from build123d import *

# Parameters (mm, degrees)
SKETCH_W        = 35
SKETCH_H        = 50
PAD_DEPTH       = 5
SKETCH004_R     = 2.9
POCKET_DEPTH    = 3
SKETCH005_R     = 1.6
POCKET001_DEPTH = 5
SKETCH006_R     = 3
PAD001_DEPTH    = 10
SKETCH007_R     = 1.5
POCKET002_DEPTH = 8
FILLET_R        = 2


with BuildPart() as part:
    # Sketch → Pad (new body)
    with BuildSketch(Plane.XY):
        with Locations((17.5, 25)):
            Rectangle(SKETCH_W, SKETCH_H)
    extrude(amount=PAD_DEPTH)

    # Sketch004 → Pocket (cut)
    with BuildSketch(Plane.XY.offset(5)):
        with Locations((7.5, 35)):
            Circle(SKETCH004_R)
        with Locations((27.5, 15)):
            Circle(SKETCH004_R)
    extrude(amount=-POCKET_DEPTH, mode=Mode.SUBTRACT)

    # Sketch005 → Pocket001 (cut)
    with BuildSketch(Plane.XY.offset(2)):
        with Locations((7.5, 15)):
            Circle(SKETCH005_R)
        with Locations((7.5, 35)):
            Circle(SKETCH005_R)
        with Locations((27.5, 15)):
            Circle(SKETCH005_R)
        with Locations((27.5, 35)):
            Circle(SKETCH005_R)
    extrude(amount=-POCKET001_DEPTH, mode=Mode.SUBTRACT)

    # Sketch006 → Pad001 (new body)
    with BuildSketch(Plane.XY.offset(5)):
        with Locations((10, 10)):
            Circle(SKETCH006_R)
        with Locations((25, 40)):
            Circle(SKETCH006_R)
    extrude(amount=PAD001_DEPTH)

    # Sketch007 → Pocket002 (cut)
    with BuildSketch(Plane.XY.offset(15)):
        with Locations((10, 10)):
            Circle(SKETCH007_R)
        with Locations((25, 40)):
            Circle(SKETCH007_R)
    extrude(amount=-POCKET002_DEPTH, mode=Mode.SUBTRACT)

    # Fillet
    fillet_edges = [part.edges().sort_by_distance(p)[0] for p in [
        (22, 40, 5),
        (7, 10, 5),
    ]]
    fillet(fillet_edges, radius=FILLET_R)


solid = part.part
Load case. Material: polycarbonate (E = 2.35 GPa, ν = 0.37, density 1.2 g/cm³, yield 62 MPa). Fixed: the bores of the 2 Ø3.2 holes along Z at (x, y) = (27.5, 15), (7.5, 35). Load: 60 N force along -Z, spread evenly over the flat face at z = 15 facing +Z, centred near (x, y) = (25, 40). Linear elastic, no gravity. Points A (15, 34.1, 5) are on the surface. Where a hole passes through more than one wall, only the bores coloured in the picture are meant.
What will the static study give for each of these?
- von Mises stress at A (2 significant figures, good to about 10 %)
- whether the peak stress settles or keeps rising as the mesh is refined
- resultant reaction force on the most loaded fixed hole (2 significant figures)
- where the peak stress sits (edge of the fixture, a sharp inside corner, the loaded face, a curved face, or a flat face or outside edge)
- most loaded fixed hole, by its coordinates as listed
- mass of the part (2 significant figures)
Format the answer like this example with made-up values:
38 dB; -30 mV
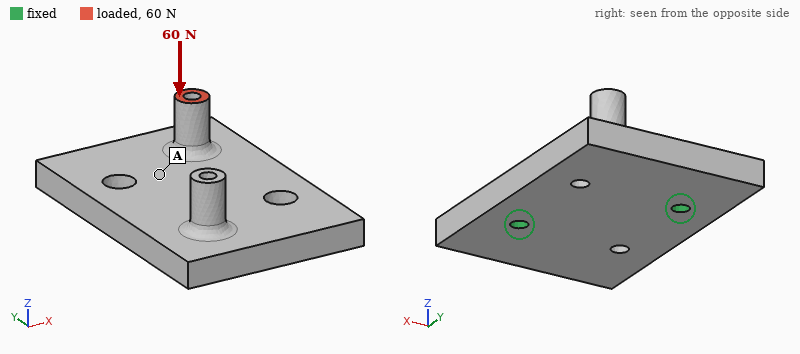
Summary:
5.0 MPa; keeps rising; 49 N; edge of the fixture; (7.5, 35); 11 g
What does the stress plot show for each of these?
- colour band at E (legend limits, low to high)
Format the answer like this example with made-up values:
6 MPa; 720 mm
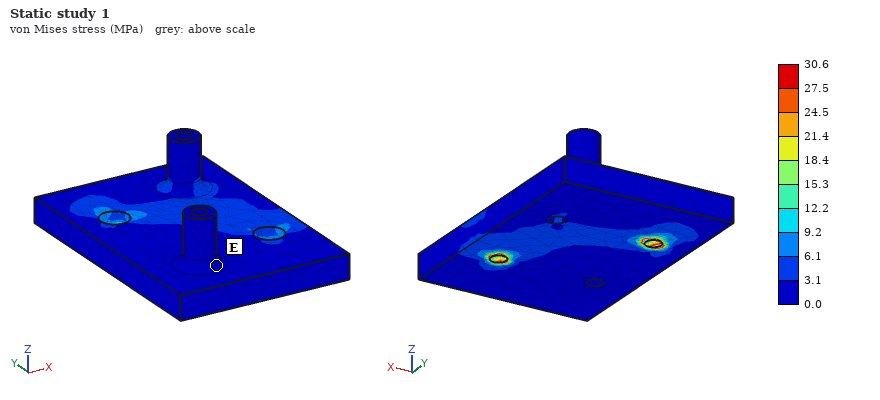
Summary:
0.0 to 3.1 MPa
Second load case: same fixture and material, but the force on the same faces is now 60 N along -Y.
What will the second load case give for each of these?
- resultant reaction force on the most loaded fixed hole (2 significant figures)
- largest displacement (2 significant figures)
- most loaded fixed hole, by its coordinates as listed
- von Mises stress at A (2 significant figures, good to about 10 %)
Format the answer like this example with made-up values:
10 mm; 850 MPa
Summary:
52 N; 0.59 mm; (27.5, 15); 5.2 MPa
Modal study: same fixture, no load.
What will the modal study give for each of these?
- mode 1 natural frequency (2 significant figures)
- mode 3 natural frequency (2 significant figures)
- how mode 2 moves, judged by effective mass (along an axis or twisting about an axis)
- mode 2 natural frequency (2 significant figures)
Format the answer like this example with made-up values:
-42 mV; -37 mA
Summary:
840 Hz; 3100 Hz; along Z; 1700 Hz
